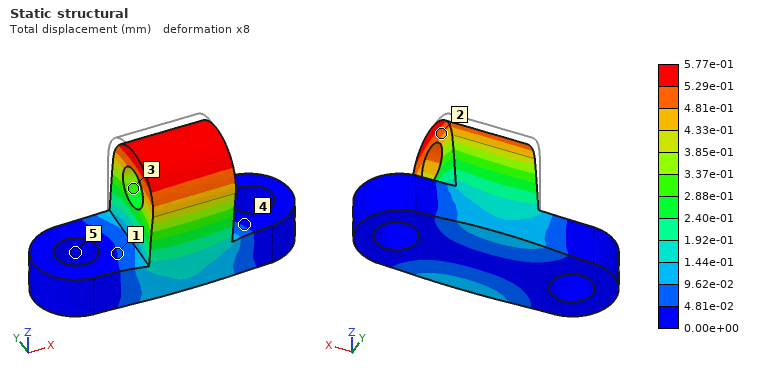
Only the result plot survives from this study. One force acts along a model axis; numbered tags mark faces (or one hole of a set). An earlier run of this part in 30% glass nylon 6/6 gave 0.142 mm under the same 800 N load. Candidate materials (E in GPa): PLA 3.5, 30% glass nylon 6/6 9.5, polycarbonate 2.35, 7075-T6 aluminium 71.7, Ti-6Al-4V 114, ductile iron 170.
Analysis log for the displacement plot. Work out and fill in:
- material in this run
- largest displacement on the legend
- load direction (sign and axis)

polycarbonate
5.77e-01 mm
-Y
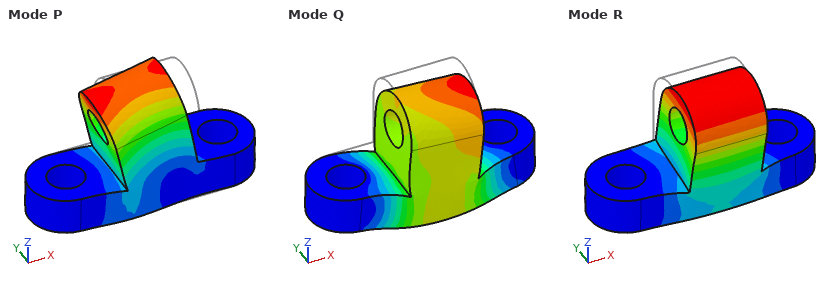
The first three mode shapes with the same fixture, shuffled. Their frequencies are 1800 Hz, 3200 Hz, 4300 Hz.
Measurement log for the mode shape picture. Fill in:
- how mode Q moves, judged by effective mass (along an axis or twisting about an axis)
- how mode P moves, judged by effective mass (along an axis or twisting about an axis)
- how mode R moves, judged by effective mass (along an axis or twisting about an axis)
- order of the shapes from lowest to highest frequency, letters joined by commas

along Z
along X
along Y
R, P, Q
